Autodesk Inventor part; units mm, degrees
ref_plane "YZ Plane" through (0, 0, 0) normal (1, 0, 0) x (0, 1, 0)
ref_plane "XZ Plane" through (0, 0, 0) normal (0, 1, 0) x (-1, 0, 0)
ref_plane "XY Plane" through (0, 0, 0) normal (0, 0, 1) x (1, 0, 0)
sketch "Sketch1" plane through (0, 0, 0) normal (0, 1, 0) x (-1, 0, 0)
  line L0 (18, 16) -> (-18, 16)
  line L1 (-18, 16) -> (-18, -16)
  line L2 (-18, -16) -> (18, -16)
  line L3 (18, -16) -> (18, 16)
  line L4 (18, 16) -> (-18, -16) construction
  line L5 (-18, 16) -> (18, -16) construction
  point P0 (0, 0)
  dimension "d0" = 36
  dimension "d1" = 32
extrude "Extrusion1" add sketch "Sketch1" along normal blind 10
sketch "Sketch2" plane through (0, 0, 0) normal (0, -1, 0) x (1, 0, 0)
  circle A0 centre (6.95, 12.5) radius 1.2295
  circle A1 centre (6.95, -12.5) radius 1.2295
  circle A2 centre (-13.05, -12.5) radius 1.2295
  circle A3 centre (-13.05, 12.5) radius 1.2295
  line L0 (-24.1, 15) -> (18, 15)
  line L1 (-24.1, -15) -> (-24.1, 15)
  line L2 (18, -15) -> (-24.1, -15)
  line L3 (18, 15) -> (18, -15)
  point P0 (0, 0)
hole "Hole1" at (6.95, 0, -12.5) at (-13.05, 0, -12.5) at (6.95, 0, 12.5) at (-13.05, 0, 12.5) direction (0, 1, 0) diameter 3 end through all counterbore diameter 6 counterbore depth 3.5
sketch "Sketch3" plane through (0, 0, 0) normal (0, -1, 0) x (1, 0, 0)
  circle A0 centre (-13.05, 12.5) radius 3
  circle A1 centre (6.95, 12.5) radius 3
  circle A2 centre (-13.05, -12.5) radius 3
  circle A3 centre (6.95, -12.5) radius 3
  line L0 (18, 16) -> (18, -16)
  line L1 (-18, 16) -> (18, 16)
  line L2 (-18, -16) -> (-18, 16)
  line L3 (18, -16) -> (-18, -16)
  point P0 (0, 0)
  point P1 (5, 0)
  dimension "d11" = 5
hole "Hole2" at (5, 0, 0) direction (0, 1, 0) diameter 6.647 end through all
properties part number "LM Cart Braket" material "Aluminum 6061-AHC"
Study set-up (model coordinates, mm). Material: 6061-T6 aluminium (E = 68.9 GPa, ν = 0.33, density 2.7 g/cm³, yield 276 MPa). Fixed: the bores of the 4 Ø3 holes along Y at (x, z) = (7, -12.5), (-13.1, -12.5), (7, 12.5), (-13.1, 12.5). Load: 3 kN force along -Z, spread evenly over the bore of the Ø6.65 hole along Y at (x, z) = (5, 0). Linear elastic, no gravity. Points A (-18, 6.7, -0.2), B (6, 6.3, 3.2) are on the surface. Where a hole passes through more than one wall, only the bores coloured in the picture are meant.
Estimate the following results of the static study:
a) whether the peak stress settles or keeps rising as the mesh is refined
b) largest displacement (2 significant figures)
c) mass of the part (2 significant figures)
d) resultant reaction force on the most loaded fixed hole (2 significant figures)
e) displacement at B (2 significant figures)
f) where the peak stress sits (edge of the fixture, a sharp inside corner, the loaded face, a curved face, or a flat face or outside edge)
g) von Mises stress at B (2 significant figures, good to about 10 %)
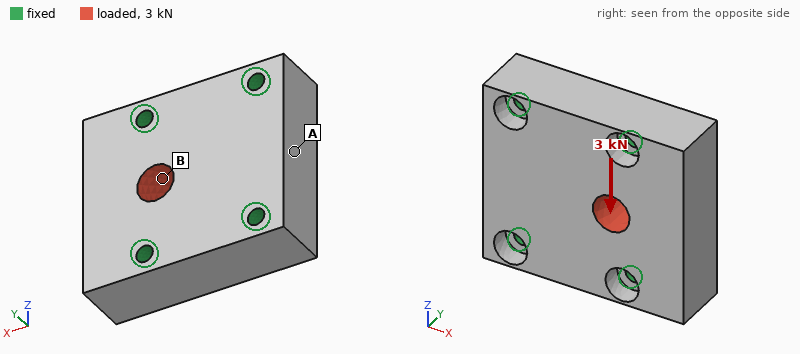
keeps rising
2.9 µm
29 g
1.2 kN
2.3 µm
edge of the fixture
16 MPa
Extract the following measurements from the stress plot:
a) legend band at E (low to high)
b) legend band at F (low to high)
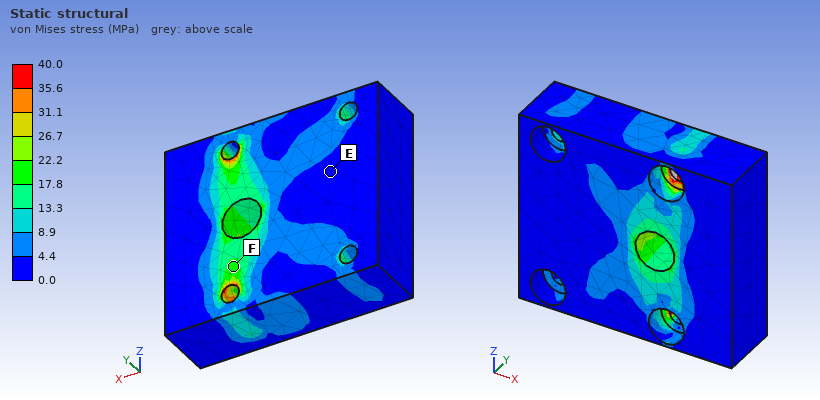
0.0 to 4.4 MPa
17.8 to 22.2 MPa
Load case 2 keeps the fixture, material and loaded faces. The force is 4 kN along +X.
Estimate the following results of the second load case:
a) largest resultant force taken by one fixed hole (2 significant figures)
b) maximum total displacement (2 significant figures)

1.2 kN
6.1 µm
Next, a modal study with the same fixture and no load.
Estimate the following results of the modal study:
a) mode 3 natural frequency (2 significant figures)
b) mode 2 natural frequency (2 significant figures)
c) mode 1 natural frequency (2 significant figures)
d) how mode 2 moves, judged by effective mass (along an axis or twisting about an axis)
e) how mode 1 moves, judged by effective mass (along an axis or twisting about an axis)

42 kHz
36 kHz
26 kHz
along Y
along Y
